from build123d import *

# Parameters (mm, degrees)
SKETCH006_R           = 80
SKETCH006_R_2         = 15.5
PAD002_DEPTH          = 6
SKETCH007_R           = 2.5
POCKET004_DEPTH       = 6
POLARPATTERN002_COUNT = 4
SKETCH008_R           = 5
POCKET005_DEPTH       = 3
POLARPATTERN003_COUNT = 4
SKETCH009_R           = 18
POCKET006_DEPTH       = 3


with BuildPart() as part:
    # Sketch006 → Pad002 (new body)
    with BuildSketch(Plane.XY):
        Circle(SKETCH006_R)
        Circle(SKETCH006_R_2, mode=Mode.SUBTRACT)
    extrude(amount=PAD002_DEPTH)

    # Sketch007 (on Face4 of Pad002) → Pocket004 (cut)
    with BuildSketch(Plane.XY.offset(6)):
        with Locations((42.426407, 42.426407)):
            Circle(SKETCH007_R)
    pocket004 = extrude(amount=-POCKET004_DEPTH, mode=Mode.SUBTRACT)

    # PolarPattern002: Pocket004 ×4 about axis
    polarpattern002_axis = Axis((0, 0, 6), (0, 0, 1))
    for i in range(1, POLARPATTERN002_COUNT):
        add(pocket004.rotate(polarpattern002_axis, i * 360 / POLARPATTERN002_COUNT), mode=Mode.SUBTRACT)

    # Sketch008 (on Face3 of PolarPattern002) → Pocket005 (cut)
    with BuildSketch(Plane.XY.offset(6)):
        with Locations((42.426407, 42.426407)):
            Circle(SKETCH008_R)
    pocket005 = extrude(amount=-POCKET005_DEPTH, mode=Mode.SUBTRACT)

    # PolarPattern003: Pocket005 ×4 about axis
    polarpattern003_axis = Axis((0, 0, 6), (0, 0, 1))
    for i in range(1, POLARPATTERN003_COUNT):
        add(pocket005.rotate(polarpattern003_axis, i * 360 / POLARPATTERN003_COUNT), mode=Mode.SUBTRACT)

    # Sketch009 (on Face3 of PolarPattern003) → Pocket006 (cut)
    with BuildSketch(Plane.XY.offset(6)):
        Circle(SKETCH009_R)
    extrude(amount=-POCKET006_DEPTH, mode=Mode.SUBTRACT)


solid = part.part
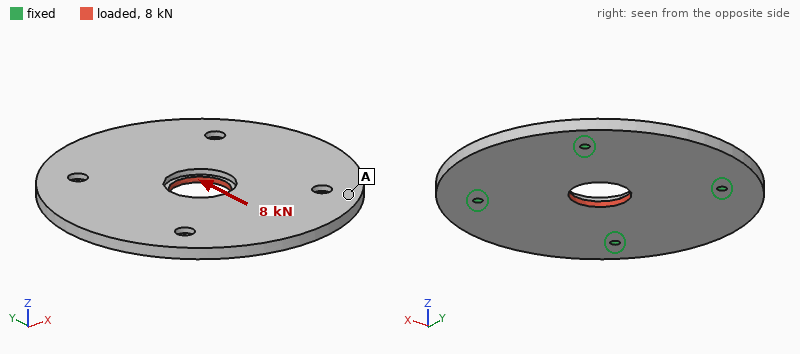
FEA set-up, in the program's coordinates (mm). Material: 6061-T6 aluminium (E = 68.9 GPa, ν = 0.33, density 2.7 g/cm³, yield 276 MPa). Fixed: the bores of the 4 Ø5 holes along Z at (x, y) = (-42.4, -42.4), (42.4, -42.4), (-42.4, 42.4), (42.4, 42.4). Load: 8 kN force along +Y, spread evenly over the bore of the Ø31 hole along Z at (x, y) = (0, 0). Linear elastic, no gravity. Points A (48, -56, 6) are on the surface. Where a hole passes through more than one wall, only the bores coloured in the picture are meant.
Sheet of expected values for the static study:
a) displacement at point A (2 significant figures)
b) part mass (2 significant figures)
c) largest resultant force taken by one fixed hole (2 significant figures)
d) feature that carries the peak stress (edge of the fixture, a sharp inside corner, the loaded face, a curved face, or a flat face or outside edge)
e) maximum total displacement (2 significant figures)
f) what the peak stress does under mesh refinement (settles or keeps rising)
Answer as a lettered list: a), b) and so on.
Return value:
a) 7.4 µm
b) 310 g
c) 2.0 kN
d) edge of the fixture
e) 16 µm
f) keeps rising
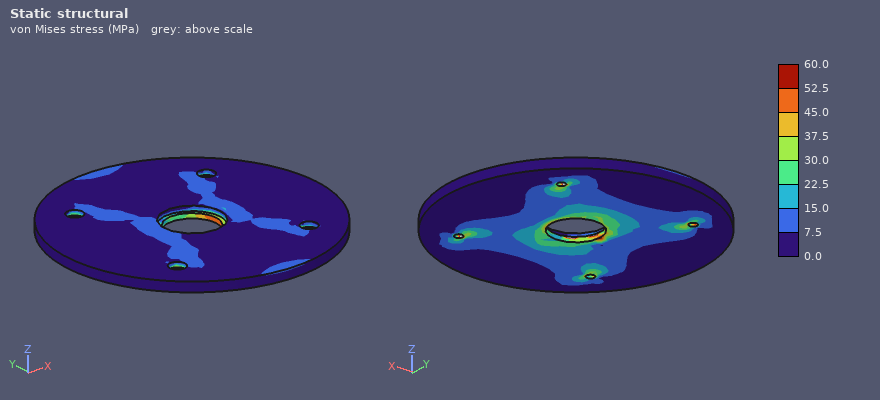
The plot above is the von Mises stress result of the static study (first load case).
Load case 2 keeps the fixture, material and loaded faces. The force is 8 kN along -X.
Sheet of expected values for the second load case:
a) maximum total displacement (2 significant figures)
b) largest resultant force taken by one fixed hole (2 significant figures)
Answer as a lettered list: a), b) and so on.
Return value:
a) 16 µm
b) 2.0 kN
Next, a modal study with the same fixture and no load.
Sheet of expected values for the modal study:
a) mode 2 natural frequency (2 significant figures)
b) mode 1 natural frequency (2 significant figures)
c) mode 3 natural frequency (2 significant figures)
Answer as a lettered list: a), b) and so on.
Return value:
a) 2300 Hz
b) 1800 Hz
c) 2300 Hz
